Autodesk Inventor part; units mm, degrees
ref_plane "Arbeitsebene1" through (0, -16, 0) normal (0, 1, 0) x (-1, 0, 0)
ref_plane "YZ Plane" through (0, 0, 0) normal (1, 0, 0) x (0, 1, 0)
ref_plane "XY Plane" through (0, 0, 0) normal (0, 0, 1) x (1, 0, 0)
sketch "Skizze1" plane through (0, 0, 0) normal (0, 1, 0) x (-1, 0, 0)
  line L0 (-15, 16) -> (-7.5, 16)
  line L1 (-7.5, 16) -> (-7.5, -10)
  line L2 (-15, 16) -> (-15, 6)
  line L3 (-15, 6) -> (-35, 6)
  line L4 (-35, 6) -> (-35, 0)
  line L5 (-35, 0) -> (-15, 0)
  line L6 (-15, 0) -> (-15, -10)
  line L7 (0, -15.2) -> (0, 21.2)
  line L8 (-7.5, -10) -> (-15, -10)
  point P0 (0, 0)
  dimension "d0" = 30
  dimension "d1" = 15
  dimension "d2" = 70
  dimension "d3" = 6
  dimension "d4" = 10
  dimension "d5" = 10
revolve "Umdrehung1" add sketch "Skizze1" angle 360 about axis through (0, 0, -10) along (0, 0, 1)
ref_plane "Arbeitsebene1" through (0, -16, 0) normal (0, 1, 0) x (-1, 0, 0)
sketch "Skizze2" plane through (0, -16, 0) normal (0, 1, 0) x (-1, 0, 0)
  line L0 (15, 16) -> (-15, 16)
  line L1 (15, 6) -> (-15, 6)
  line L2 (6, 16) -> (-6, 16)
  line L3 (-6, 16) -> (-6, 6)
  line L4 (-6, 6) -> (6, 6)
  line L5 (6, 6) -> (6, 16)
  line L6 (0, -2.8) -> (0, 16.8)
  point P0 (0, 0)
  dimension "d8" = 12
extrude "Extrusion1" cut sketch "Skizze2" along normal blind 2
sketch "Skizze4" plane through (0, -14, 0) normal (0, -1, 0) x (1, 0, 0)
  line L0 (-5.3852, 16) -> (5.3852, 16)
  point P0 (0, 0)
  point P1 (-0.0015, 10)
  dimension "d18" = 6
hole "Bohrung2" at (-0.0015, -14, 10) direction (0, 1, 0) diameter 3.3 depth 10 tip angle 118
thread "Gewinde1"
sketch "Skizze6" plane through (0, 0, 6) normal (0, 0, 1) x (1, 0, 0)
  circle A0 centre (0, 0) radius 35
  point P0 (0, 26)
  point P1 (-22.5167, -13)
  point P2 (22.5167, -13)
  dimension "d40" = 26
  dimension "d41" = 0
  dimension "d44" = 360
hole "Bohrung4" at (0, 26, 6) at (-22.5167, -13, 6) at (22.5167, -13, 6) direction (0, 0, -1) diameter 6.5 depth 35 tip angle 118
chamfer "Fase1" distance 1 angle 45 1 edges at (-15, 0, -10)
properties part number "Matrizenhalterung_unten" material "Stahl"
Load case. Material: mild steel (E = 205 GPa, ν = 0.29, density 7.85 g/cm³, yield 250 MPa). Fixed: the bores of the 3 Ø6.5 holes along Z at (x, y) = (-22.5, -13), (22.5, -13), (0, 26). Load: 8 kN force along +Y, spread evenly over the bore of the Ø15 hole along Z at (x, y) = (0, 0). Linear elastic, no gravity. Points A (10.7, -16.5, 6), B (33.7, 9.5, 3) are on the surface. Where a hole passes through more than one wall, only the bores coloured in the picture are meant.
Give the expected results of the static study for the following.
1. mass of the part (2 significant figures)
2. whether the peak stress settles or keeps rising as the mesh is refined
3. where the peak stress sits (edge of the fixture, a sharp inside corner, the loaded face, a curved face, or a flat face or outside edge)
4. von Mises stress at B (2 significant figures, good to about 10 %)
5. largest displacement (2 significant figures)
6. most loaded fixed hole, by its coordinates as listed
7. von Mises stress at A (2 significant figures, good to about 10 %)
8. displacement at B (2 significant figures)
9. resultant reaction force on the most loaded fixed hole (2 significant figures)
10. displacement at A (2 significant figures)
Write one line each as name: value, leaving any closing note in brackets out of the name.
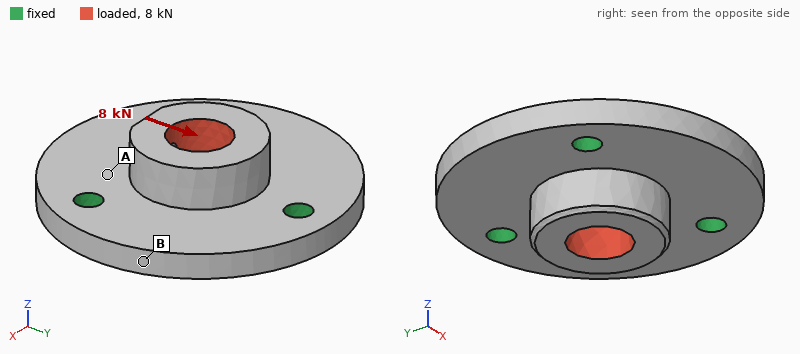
mass of the part: 250 g
whether the peak stress settles or keeps rising as the mesh is refined: keeps rising
where the peak stress sits: edge of the fixture
von Mises stress at B: 4.6 MPa
largest displacement: 3.6 µm
most loaded fixed hole, by its coordinates as listed: (0, 26)
von Mises stress at A: 14 MPa
displacement at B: 0.67 µm
resultant reaction force on the most loaded fixed hole: 2.9 kN
displacement at A: 1.7 µm
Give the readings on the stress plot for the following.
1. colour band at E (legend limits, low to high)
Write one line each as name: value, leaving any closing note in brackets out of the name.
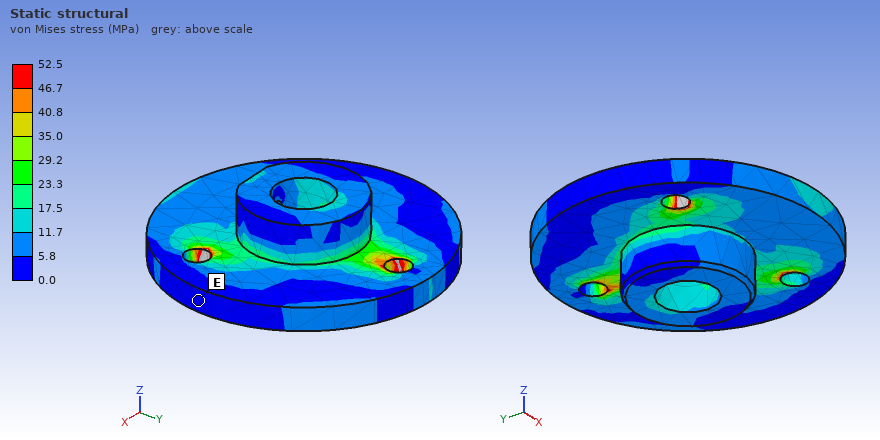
colour band at E: 0.0 to 5.8 MPa
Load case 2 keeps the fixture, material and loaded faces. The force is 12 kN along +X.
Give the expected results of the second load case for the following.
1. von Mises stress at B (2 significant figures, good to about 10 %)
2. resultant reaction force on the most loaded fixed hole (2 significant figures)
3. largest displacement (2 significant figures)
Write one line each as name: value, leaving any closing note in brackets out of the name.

von Mises stress at B: 16 MPa
resultant reaction force on the most loaded fixed hole: 4.2 kN
largest displacement: 5.1 µm
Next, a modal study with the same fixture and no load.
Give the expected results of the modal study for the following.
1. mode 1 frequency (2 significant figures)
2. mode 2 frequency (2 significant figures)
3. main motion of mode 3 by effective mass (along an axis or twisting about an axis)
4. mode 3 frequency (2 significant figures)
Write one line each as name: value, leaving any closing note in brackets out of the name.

mode 1 frequency: 10 kHz
mode 2 frequency: 10 kHz
main motion of mode 3 by effective mass: along Z
mode 3 frequency: 11 kHz
